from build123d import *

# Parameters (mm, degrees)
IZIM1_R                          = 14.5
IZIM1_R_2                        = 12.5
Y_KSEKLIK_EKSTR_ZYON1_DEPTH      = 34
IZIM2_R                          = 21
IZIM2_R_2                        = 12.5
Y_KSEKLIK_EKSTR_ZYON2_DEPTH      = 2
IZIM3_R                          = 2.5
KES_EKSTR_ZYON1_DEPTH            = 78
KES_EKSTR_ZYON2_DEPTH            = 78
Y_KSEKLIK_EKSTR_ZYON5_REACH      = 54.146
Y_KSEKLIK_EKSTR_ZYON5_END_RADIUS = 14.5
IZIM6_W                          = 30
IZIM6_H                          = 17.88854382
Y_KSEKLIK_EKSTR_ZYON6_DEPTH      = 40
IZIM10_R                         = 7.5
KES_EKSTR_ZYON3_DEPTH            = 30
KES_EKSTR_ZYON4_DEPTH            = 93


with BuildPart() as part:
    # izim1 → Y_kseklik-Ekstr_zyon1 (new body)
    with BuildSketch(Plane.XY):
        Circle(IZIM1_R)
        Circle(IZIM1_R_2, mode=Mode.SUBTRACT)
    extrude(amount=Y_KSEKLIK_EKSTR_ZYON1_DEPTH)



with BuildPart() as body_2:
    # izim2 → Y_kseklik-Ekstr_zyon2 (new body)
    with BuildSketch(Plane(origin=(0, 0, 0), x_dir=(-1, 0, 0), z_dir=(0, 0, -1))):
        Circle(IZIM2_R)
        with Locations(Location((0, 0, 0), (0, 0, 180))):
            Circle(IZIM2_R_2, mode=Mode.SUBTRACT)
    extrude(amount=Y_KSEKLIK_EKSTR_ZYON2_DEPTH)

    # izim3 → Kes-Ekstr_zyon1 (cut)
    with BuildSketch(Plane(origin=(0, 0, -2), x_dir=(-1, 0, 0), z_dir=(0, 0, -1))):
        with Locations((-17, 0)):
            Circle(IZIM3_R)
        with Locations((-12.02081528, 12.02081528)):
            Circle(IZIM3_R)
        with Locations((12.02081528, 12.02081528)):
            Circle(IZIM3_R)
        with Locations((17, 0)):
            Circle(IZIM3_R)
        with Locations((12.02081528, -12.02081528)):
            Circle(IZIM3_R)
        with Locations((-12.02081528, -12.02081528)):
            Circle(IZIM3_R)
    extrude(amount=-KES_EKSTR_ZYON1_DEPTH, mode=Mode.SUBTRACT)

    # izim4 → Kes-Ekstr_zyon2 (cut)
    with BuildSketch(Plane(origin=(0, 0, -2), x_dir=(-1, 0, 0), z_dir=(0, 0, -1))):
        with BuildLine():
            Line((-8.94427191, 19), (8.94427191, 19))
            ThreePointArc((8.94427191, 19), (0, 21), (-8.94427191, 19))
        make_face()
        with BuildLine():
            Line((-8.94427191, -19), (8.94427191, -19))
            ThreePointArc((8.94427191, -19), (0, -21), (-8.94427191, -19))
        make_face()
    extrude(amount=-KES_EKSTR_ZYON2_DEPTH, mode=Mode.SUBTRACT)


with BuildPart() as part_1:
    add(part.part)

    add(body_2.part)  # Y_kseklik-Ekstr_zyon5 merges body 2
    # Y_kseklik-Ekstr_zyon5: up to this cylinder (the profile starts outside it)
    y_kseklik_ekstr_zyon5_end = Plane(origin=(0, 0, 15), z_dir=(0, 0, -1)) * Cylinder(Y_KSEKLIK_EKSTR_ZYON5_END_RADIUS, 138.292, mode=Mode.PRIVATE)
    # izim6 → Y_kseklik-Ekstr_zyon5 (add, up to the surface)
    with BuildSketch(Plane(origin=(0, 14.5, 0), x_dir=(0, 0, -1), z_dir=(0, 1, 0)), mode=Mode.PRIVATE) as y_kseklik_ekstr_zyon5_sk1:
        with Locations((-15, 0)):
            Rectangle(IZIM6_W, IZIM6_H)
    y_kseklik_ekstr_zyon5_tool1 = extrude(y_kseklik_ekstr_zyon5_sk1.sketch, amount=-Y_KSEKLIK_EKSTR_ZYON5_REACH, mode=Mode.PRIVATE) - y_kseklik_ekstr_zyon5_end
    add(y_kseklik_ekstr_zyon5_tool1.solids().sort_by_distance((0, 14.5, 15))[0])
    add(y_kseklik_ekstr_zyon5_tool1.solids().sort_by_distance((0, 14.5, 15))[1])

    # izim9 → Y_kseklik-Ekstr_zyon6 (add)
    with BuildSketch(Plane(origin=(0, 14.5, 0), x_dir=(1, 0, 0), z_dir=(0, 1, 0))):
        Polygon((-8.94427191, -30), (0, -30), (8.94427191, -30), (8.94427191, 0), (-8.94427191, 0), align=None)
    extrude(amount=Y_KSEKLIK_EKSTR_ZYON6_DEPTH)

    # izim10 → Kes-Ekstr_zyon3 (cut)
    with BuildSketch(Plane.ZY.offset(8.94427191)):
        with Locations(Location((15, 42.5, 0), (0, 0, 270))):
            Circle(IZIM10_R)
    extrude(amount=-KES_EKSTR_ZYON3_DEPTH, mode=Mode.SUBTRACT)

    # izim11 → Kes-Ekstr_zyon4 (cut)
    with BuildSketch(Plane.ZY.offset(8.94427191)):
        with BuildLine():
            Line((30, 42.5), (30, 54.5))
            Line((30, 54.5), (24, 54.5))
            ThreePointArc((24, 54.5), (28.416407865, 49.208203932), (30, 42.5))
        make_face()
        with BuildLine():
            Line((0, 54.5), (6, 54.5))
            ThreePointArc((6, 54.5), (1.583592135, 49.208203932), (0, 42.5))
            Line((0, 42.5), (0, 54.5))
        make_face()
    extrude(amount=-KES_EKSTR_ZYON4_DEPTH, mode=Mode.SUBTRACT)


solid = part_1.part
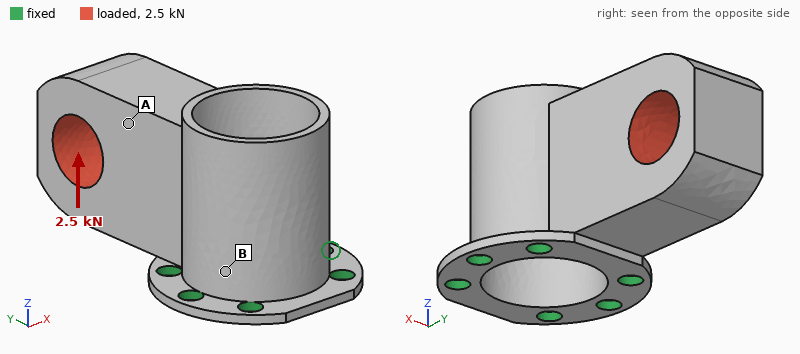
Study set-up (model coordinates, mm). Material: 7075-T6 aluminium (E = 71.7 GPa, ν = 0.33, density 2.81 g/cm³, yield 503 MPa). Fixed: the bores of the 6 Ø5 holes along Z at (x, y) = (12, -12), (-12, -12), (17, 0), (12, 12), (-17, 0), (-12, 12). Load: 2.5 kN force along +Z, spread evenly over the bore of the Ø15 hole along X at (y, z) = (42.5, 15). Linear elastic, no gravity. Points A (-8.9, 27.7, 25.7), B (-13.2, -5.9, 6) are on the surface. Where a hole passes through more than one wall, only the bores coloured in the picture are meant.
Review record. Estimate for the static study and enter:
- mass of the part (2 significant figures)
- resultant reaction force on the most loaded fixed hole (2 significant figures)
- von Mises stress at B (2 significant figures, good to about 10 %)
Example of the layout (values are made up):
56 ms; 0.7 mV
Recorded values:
71 g; 3.5 kN; 75 MPa
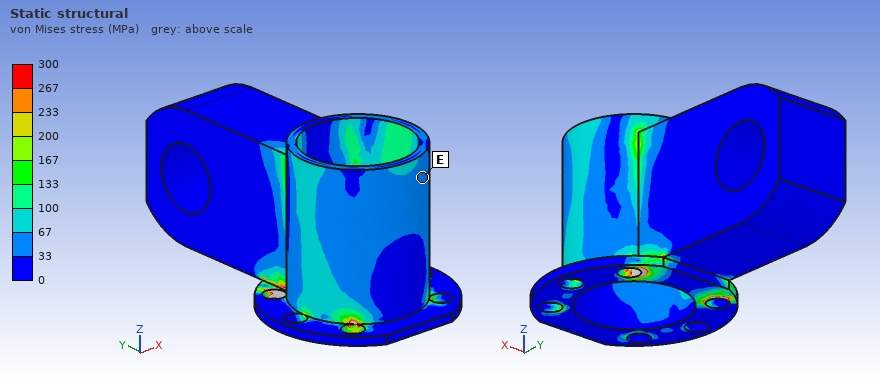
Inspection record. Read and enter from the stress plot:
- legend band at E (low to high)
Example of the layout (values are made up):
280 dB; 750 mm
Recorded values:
33 to 67 MPa
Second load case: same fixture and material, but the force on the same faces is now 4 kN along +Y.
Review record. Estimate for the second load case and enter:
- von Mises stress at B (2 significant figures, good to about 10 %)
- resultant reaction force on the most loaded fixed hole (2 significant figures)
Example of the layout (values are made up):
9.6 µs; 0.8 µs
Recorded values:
59 MPa; 1.9 kN
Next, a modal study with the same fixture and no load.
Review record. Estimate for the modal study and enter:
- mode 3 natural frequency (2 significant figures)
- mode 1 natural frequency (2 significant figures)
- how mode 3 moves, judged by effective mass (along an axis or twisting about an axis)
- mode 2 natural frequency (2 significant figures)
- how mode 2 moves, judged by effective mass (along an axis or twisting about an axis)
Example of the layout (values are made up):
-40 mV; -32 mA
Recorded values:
7600 Hz; 3000 Hz; along X; 4100 Hz; along X
